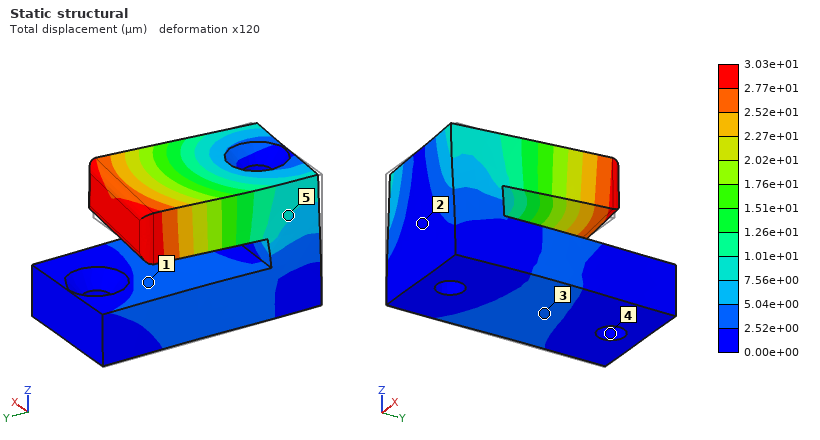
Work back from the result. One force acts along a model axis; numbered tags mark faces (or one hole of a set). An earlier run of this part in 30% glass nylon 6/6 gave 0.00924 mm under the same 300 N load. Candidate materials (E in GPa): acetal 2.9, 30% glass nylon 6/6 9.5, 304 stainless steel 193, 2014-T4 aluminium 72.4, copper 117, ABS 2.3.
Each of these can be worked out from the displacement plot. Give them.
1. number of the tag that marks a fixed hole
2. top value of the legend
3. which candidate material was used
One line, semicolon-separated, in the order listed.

4; 3.03e+01 µm; acetal
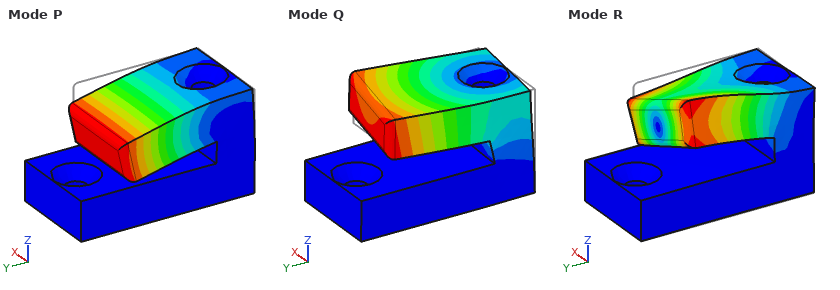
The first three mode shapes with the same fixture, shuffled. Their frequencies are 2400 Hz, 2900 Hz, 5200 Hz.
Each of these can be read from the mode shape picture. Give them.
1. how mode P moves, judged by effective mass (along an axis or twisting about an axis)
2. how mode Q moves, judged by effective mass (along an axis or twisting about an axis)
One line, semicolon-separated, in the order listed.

along Z; along X
